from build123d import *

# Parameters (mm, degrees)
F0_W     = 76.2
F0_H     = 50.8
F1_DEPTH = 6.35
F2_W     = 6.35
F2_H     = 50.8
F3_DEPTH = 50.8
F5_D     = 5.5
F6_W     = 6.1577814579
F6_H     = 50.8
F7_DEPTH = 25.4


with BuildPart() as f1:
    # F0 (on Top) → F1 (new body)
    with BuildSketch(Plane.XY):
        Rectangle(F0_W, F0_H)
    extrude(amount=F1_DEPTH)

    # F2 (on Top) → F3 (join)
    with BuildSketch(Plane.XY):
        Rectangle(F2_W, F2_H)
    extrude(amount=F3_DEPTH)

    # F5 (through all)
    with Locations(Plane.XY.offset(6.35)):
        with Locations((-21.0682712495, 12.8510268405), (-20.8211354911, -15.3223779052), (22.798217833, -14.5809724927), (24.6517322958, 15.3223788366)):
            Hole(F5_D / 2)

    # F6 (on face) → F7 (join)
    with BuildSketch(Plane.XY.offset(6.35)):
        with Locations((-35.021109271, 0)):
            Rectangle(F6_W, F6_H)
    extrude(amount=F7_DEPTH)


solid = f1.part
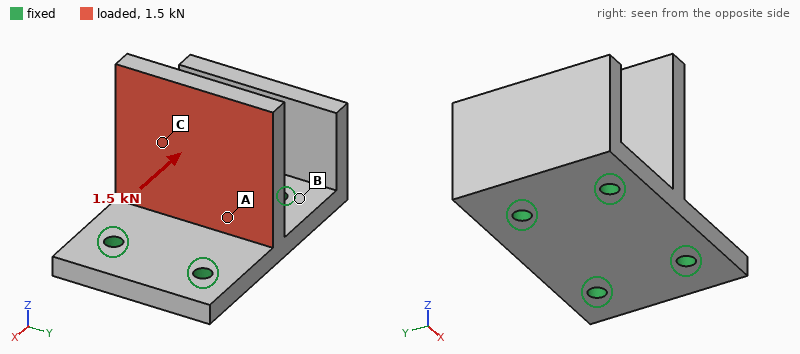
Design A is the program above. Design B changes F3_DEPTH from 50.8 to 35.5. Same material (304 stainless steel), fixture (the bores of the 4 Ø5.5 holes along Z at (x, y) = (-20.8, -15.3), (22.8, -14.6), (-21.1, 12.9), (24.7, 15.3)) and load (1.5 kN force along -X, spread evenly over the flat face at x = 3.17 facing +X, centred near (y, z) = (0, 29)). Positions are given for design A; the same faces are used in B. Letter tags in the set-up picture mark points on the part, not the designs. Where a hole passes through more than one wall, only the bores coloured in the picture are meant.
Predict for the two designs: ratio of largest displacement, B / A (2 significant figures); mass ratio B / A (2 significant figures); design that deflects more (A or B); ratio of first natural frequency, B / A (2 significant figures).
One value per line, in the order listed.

0.34
0.89
A
1.6
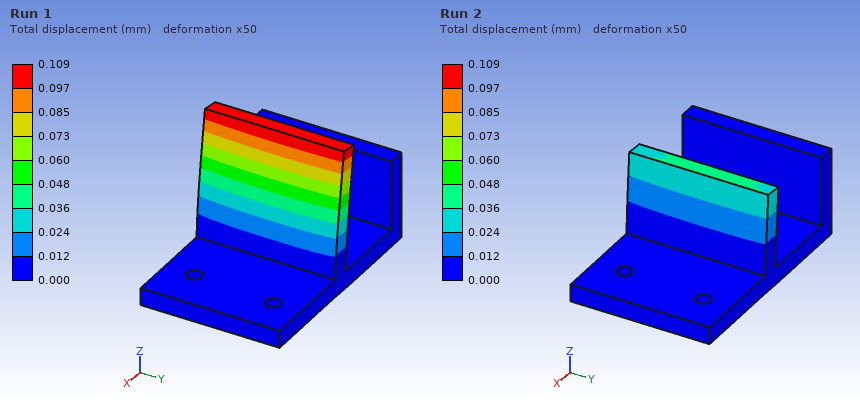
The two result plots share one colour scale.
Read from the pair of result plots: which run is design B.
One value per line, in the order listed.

Run 2
